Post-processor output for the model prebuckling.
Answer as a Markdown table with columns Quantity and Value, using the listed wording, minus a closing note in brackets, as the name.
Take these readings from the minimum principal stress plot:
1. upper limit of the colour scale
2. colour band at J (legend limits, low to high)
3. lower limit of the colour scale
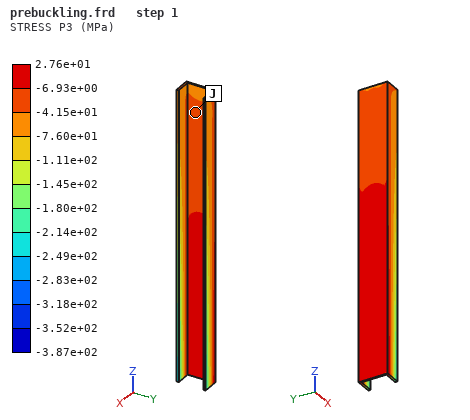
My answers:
| Quantity | Value |
|---|---|
| upper limit of the colour scale | 2.76e+01 MPa |
| colour band at J | -4.15e+01 to -6.93e+00 MPa |
| lower limit of the colour scale | -3.87e+02 MPa |
